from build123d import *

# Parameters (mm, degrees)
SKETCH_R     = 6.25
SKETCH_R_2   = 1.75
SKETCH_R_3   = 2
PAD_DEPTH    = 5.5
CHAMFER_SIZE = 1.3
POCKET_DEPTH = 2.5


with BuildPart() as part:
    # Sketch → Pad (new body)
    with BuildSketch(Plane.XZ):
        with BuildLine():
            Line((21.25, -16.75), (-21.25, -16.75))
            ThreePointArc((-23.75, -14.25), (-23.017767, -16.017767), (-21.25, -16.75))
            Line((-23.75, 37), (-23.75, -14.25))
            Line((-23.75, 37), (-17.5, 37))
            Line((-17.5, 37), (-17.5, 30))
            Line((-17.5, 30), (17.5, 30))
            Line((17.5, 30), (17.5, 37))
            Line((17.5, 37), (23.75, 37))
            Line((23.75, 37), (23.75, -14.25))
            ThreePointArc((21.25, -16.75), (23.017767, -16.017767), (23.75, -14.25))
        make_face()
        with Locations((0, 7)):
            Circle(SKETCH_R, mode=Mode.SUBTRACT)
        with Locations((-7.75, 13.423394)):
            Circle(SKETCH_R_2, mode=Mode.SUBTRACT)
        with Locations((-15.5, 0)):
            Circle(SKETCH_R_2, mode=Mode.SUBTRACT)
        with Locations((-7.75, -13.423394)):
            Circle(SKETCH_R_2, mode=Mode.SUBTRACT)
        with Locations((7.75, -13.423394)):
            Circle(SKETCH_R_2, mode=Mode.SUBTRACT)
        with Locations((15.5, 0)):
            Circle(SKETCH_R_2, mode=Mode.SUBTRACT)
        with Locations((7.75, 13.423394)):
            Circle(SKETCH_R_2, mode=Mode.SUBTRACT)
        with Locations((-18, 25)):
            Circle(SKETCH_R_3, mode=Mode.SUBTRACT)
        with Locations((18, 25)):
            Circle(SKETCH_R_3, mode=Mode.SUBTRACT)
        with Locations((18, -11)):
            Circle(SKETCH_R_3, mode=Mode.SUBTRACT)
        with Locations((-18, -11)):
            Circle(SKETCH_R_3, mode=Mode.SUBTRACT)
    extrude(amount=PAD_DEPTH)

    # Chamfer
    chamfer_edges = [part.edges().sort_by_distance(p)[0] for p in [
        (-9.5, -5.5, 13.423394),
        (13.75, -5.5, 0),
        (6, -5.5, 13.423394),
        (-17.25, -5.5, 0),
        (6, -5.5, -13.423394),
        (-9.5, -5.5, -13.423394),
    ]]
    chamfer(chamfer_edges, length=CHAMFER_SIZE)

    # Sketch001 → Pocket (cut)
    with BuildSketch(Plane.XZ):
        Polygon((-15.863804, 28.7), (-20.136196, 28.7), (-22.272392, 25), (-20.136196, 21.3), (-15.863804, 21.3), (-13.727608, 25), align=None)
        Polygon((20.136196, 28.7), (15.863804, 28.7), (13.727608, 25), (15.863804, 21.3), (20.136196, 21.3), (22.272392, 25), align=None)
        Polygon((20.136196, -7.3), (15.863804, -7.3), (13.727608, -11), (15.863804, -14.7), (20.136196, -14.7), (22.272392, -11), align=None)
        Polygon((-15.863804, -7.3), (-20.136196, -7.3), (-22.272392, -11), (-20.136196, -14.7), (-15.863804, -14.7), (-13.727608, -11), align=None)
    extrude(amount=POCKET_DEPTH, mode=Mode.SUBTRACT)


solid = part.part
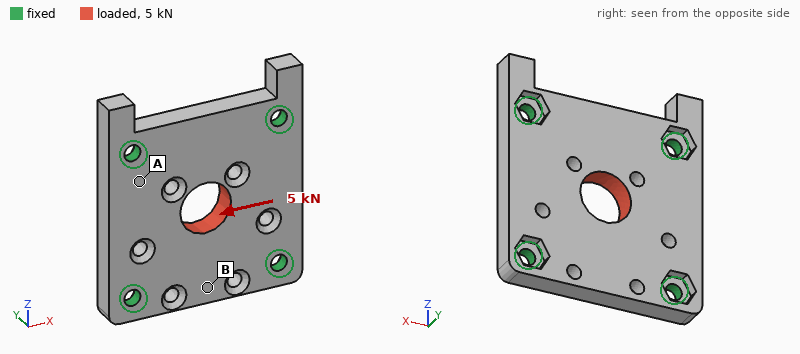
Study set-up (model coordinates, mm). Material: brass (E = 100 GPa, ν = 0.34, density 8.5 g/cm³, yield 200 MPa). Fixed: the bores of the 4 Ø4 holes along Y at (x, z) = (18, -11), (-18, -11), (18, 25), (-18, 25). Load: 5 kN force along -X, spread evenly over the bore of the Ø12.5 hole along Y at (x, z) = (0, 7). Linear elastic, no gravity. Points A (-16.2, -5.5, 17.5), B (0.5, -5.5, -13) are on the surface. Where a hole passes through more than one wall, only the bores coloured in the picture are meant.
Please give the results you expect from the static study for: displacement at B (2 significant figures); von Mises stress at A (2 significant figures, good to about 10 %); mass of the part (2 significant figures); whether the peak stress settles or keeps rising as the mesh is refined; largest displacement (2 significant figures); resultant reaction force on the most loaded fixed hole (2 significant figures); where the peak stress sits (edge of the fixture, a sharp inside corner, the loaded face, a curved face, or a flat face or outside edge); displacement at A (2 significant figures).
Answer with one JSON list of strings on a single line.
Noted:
["2.6 µm", "20 MPa", "93 g", "keeps rising", "8.2 µm", "1.4 kN", "edge of the fixture", "3.3 µm"]
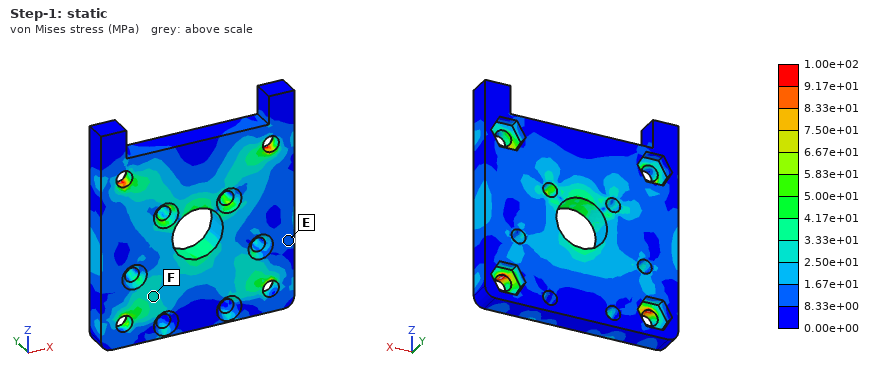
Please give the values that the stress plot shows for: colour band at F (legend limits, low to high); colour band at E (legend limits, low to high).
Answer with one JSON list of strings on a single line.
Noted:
["2.50e+01 to 3.33e+01 MPa", "8.33e+00 to 1.67e+01 MPa"]
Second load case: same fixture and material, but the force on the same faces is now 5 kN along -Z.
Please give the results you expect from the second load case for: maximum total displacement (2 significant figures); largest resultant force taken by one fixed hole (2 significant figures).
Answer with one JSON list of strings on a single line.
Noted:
["7.9 µm", "1.4 kN"]
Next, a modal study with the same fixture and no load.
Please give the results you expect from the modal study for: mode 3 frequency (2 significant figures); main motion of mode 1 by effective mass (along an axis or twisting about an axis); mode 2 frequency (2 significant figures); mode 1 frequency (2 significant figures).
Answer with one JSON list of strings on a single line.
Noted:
["12 kHz", "along Y", "12 kHz", "8100 Hz"]
